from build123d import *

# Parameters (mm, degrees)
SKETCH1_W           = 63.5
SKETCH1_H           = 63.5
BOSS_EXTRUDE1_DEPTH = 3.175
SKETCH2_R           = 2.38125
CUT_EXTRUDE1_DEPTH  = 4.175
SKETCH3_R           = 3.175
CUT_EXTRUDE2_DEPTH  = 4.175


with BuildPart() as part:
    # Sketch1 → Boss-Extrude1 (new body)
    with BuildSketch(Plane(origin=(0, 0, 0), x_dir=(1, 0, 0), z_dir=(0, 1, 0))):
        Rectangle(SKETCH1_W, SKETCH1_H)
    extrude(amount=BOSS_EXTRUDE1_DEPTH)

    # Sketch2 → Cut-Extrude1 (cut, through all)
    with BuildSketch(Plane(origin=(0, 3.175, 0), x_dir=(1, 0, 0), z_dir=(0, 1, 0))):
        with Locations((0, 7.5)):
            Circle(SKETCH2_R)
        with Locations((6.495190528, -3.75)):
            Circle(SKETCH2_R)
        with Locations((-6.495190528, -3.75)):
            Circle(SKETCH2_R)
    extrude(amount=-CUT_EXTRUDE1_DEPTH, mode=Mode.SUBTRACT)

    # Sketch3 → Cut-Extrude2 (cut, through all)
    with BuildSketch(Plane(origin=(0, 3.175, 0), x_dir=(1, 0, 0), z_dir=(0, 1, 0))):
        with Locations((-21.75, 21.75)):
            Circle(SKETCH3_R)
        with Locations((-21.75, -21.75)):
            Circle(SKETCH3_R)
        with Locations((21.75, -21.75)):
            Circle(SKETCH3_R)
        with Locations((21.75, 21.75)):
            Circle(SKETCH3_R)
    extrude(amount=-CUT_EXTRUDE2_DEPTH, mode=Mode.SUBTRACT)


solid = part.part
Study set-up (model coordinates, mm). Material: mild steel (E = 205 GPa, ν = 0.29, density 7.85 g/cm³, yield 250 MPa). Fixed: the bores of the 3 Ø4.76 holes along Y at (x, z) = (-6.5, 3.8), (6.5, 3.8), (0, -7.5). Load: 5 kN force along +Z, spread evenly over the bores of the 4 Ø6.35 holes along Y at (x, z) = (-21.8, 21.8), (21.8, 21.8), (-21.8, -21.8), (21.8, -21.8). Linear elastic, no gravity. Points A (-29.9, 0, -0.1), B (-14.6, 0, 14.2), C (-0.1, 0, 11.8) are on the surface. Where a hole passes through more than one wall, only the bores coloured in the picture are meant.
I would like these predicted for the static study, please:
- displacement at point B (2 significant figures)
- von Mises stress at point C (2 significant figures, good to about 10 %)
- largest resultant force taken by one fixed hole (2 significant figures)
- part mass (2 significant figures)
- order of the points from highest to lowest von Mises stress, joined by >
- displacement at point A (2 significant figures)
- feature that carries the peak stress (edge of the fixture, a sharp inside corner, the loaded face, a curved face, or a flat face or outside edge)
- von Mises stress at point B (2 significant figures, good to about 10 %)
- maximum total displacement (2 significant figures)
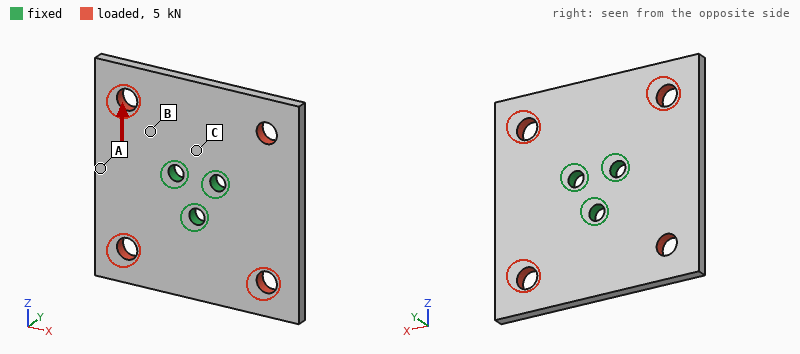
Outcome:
2.5 µm
13 MPa
1.8 kN
96 g
B > C > A
4.5 µm
edge of the fixture
28 MPa
5.7 µm
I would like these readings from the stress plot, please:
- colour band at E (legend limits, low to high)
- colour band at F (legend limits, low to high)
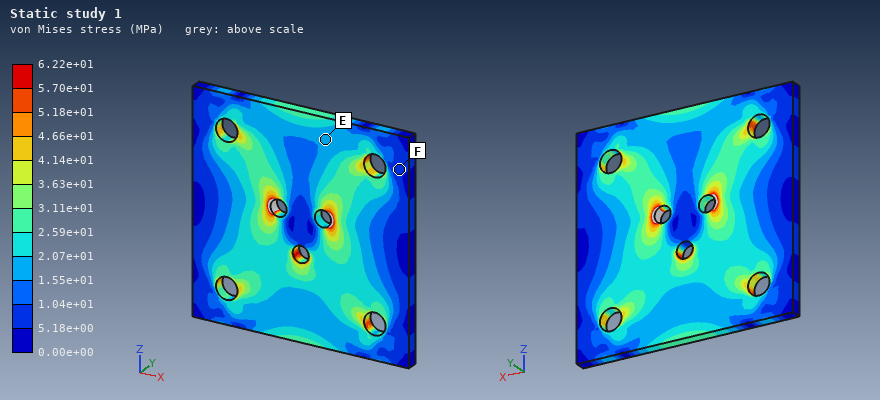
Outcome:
1.55e+01 to 2.07e+01 MPa
5.18e+00 to 1.04e+01 MPa
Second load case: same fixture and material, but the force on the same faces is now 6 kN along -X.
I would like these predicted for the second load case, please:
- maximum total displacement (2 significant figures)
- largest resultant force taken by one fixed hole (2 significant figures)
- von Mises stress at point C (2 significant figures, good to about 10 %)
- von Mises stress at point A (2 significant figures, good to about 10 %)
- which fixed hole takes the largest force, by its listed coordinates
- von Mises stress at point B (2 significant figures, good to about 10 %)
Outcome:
7.1 µm
2.3 kN
37 MPa
30 MPa
(0, -7.5)
32 MPa
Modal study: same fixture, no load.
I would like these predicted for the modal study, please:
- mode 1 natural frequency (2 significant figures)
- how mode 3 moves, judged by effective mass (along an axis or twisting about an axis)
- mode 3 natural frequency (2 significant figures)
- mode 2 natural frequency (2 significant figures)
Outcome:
2700 Hz
along Y
3100 Hz
2800 Hz
